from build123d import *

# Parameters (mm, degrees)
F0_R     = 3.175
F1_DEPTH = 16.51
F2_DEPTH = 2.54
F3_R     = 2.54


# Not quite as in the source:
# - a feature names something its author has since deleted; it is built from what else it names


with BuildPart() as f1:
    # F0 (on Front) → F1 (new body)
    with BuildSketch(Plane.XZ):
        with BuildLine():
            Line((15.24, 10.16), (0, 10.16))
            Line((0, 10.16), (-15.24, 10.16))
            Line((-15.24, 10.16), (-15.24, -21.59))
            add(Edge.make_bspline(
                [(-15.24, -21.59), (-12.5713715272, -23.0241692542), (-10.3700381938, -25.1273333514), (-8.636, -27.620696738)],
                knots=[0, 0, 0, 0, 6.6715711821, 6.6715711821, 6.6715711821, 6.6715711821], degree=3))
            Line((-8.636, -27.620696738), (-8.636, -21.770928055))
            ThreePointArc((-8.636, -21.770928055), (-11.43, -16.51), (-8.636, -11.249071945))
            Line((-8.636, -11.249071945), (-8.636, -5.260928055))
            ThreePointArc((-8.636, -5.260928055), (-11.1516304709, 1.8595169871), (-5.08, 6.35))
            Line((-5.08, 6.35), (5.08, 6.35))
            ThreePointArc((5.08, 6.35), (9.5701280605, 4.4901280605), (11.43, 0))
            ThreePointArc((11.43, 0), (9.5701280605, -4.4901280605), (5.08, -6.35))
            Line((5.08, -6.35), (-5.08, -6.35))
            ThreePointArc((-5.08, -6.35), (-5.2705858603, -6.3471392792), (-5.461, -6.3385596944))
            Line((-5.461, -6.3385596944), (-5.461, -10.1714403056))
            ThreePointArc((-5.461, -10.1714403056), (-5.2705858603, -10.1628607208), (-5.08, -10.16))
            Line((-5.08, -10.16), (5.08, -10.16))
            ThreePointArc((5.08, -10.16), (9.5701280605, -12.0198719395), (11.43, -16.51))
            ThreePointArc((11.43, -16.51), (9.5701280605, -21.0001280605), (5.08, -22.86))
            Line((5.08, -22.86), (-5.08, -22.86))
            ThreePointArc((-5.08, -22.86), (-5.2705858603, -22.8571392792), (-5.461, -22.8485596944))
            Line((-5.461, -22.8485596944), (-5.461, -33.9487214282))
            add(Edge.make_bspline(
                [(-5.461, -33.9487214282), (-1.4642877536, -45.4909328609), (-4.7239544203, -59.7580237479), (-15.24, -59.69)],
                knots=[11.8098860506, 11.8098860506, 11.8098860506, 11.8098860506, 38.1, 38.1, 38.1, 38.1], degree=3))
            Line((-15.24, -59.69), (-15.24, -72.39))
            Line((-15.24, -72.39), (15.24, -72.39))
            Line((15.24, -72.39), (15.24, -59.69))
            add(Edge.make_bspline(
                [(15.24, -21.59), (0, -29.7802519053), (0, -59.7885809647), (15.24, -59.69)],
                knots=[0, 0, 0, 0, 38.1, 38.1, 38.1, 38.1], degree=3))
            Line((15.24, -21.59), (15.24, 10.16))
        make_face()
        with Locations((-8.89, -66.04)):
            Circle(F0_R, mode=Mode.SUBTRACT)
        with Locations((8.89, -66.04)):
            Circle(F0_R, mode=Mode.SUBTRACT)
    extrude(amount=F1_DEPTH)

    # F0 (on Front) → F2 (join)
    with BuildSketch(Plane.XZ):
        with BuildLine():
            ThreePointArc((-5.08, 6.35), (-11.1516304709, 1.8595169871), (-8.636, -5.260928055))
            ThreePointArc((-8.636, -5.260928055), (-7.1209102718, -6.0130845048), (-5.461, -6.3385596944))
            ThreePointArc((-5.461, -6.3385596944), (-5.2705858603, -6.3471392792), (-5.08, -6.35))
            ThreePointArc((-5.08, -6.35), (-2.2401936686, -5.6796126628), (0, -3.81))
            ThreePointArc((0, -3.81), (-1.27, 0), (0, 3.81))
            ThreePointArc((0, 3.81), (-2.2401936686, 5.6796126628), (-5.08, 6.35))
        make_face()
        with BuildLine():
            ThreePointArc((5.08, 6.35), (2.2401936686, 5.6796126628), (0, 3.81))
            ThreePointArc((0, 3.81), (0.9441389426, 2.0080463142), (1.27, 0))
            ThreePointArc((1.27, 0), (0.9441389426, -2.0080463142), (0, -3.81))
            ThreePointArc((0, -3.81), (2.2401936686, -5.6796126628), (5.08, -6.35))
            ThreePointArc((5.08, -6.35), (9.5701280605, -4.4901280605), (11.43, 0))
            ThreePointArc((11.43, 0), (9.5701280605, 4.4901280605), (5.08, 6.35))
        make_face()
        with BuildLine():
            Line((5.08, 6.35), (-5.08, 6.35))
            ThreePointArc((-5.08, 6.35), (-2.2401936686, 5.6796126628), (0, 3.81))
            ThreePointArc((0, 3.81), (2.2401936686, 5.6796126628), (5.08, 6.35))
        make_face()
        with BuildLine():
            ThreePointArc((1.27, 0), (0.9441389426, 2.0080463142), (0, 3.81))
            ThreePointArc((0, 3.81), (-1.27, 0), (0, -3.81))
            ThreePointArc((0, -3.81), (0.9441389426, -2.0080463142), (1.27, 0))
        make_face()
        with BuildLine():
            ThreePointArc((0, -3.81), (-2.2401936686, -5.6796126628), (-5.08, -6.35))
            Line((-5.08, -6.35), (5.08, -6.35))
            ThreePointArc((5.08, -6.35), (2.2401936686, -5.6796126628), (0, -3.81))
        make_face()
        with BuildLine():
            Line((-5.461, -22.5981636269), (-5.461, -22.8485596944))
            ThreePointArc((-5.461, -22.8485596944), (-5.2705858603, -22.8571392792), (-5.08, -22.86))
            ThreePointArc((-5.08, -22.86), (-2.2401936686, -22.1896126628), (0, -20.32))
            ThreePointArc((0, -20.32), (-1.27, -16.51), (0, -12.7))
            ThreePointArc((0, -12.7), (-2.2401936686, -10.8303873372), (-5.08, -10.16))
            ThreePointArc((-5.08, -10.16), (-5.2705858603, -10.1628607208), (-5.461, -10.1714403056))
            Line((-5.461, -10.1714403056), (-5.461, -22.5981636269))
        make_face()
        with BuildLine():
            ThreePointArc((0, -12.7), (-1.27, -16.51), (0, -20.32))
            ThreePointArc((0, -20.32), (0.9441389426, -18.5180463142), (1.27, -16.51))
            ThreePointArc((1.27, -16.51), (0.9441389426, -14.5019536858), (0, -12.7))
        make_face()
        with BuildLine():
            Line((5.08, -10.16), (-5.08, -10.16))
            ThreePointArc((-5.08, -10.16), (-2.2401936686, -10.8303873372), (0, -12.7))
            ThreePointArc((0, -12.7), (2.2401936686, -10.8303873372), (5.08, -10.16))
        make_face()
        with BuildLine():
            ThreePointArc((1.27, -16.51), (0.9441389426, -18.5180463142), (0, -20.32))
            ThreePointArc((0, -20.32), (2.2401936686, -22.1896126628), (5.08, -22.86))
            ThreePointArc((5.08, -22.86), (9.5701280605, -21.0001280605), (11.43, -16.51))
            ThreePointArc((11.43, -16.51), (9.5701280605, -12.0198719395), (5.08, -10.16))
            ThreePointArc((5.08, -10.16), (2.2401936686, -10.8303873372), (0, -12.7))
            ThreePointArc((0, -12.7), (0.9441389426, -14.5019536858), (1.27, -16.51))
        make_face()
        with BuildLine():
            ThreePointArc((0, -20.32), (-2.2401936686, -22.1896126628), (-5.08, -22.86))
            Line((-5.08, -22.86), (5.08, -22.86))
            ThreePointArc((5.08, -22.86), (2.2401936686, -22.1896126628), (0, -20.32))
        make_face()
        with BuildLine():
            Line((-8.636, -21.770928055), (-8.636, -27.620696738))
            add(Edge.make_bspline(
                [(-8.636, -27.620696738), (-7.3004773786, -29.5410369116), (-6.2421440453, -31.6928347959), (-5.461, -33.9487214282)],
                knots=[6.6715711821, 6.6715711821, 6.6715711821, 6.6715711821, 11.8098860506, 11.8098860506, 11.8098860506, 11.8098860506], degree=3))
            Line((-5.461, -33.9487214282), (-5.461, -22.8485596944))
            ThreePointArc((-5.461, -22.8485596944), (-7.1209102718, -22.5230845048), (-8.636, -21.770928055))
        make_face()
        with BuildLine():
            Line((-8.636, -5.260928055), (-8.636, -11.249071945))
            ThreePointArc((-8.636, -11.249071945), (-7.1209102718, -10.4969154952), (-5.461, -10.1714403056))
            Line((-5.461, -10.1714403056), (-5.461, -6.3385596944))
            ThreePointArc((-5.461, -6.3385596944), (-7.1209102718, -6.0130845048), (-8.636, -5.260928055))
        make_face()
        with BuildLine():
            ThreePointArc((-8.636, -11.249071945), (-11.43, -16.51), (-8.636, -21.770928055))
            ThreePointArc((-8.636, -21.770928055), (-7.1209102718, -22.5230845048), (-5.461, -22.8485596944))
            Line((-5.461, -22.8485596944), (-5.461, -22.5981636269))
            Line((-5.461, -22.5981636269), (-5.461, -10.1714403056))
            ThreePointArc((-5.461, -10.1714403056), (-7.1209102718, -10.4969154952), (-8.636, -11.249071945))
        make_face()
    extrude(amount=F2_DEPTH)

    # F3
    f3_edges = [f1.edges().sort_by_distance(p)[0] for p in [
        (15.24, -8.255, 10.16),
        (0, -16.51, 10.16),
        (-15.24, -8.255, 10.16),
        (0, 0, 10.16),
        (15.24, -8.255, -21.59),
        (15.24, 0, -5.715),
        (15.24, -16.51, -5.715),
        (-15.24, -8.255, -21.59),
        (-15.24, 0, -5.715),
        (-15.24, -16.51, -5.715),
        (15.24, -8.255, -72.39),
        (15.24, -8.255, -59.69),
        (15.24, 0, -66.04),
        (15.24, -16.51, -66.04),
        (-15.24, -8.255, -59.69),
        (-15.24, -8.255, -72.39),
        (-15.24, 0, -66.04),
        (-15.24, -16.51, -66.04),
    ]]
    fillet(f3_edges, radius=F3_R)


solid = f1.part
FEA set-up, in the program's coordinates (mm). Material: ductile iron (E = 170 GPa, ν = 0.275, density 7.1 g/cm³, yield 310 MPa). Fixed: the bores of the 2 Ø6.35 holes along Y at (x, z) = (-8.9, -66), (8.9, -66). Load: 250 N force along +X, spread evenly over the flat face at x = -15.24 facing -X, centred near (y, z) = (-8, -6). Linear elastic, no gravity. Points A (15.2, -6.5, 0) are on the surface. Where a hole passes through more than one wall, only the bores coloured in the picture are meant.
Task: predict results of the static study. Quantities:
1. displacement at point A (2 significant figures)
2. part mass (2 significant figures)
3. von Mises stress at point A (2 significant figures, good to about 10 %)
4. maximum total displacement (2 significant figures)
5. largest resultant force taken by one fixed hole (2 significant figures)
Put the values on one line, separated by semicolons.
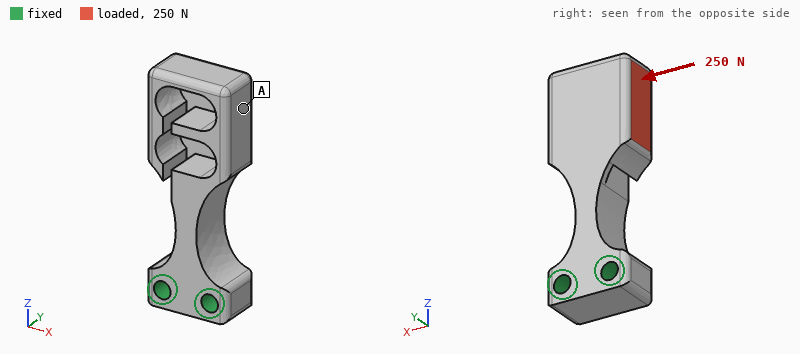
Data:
81 µm; 150 g; 8.2 MPa; 100 µm; 830 N
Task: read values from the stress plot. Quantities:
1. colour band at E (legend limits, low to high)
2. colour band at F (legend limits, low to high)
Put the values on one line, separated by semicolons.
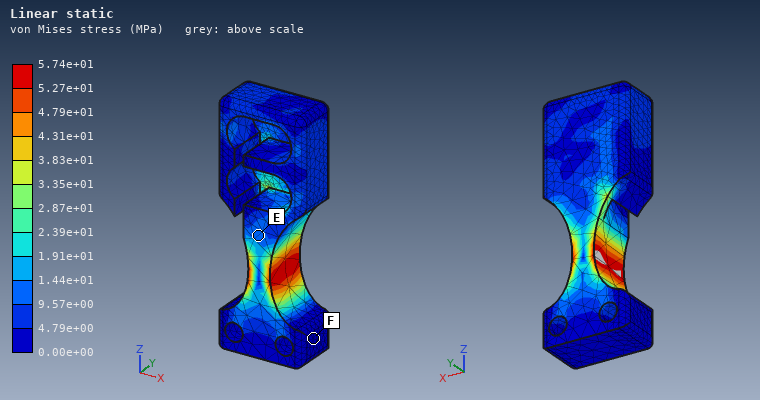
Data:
9.57e+00 to 1.44e+01 MPa; 0.00e+00 to 4.79e+00 MPa
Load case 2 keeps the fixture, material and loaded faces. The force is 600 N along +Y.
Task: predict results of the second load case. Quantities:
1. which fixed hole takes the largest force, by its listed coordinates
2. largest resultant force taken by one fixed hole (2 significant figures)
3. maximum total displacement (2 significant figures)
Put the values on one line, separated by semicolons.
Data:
(-8.9, -66); 660 N; 0.24 mm
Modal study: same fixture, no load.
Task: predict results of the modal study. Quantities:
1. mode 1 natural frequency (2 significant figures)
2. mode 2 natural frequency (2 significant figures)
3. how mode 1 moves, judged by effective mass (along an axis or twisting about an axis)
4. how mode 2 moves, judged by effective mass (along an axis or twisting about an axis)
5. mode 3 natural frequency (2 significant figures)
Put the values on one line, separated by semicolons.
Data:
1100 Hz; 1400 Hz; along X; along Y; 3300 Hz
